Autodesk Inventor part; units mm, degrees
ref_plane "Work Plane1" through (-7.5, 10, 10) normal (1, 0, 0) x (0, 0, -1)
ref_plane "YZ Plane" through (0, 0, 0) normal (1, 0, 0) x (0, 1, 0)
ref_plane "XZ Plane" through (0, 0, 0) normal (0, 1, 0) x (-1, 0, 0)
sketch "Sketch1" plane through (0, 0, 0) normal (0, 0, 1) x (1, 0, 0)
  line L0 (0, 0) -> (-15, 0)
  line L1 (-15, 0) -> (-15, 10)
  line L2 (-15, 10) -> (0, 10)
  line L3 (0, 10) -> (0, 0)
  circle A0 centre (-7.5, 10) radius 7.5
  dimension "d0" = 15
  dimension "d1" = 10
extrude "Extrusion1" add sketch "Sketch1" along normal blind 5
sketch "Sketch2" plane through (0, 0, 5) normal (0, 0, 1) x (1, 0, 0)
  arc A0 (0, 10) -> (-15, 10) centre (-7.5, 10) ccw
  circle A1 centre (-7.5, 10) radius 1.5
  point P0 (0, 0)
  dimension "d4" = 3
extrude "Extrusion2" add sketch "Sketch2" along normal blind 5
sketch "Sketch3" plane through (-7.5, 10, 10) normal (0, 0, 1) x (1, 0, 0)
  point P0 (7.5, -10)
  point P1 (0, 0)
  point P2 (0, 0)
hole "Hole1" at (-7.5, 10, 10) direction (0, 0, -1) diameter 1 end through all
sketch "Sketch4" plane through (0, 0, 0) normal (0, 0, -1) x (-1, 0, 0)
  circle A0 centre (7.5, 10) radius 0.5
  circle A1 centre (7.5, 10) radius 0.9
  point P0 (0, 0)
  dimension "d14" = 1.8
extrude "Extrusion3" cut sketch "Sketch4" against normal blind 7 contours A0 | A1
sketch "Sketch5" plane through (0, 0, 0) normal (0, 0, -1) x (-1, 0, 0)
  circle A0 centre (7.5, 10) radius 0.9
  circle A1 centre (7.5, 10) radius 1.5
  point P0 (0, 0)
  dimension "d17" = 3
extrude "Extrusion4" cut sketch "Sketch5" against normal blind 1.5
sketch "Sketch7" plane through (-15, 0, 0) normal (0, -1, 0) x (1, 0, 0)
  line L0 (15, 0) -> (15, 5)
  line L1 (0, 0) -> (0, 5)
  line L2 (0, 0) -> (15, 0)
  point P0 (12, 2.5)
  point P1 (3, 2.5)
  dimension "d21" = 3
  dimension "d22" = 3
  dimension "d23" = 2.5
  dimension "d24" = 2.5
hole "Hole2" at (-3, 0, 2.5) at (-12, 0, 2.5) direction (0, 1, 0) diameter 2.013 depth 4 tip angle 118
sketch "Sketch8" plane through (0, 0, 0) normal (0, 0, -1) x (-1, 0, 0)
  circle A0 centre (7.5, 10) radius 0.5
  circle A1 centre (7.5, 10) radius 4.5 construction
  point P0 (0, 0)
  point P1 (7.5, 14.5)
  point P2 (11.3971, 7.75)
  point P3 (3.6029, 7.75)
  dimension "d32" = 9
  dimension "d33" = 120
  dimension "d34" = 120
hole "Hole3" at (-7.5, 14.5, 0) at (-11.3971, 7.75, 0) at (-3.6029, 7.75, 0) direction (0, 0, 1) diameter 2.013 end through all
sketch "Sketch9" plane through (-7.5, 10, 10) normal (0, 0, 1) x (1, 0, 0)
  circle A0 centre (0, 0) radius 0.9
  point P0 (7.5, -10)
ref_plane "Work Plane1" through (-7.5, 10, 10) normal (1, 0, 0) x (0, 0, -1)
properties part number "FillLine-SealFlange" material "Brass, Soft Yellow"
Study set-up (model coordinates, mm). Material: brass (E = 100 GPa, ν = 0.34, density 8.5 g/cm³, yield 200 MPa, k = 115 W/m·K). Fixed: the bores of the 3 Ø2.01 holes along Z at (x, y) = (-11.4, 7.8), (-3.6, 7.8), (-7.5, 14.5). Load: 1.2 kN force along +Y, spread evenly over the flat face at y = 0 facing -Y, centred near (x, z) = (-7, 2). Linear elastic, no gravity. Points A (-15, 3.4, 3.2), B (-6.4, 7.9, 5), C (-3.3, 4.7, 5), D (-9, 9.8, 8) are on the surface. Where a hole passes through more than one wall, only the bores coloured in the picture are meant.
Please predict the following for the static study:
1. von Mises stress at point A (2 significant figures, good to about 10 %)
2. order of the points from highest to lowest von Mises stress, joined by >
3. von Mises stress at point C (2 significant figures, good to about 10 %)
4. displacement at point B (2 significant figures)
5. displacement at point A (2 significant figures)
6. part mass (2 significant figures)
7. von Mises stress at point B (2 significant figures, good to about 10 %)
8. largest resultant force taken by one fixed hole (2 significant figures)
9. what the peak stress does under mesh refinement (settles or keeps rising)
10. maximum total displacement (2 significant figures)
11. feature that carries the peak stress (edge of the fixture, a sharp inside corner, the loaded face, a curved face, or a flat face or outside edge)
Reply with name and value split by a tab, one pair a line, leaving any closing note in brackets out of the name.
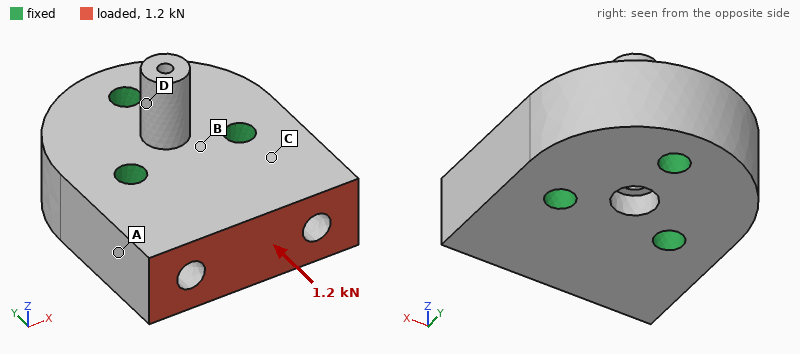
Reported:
von Mises stress at point A	14 MPa
order of the points from highest to lowest von Mises stress, joined by >	C > A > B > D
von Mises stress at point C	21 MPa
displacement at point B	0.34 µm
displacement at point A	1.1 µm
part mass	9.6 g
von Mises stress at point B	8.4 MPa
largest resultant force taken by one fixed hole	570 N
what the peak stress does under mesh refinement	keeps rising
maximum total displacement	1.6 µm
feature that carries the peak stress	edge of the fixture
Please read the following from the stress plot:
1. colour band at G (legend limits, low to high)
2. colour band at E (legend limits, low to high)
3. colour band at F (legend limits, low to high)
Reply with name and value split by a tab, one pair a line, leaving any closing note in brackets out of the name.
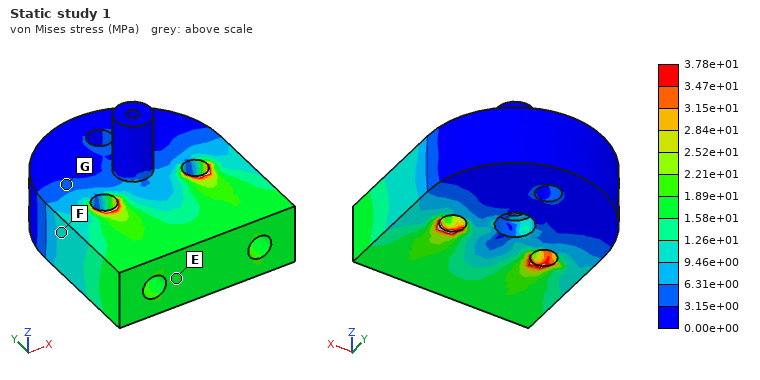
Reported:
colour band at G	3.15e+00 to 6.31e+00 MPa
colour band at E	1.58e+01 to 1.89e+01 MPa
colour band at F	9.46e+00 to 1.26e+01 MPa
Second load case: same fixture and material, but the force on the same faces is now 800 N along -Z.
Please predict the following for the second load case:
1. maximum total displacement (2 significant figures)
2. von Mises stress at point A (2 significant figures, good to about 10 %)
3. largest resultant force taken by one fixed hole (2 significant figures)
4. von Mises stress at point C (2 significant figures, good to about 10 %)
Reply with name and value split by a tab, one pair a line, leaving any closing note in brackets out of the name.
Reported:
maximum total displacement	12 µm
von Mises stress at point A	29 MPa
largest resultant force taken by one fixed hole	460 N
von Mises stress at point C	70 MPa
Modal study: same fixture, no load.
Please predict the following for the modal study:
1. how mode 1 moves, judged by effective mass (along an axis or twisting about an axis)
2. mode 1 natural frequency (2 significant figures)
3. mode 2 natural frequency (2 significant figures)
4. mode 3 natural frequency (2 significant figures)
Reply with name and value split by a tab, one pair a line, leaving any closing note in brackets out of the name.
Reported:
how mode 1 moves, judged by effective mass	along Z
mode 1 natural frequency	36 kHz
mode 2 natural frequency	38 kHz
mode 3 natural frequency	38 kHz
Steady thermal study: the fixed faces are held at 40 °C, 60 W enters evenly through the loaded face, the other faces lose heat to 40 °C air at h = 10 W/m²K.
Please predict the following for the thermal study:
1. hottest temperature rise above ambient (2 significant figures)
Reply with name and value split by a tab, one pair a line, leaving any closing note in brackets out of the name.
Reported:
hottest temperature rise above ambient	57 K
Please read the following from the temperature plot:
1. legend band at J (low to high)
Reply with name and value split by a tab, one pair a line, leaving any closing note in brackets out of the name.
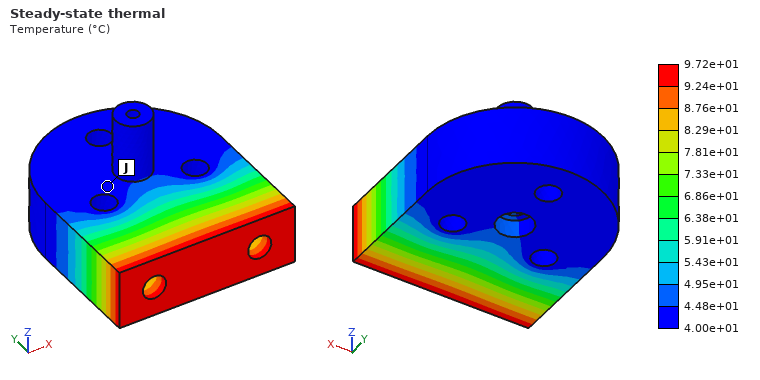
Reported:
legend band at J	4.00e+01 to 4.48e+01 °C
